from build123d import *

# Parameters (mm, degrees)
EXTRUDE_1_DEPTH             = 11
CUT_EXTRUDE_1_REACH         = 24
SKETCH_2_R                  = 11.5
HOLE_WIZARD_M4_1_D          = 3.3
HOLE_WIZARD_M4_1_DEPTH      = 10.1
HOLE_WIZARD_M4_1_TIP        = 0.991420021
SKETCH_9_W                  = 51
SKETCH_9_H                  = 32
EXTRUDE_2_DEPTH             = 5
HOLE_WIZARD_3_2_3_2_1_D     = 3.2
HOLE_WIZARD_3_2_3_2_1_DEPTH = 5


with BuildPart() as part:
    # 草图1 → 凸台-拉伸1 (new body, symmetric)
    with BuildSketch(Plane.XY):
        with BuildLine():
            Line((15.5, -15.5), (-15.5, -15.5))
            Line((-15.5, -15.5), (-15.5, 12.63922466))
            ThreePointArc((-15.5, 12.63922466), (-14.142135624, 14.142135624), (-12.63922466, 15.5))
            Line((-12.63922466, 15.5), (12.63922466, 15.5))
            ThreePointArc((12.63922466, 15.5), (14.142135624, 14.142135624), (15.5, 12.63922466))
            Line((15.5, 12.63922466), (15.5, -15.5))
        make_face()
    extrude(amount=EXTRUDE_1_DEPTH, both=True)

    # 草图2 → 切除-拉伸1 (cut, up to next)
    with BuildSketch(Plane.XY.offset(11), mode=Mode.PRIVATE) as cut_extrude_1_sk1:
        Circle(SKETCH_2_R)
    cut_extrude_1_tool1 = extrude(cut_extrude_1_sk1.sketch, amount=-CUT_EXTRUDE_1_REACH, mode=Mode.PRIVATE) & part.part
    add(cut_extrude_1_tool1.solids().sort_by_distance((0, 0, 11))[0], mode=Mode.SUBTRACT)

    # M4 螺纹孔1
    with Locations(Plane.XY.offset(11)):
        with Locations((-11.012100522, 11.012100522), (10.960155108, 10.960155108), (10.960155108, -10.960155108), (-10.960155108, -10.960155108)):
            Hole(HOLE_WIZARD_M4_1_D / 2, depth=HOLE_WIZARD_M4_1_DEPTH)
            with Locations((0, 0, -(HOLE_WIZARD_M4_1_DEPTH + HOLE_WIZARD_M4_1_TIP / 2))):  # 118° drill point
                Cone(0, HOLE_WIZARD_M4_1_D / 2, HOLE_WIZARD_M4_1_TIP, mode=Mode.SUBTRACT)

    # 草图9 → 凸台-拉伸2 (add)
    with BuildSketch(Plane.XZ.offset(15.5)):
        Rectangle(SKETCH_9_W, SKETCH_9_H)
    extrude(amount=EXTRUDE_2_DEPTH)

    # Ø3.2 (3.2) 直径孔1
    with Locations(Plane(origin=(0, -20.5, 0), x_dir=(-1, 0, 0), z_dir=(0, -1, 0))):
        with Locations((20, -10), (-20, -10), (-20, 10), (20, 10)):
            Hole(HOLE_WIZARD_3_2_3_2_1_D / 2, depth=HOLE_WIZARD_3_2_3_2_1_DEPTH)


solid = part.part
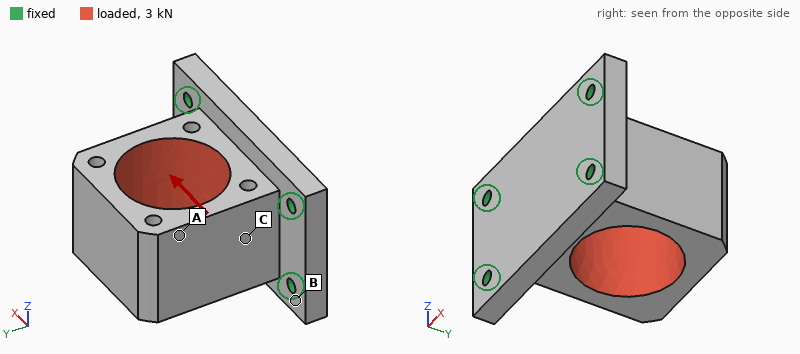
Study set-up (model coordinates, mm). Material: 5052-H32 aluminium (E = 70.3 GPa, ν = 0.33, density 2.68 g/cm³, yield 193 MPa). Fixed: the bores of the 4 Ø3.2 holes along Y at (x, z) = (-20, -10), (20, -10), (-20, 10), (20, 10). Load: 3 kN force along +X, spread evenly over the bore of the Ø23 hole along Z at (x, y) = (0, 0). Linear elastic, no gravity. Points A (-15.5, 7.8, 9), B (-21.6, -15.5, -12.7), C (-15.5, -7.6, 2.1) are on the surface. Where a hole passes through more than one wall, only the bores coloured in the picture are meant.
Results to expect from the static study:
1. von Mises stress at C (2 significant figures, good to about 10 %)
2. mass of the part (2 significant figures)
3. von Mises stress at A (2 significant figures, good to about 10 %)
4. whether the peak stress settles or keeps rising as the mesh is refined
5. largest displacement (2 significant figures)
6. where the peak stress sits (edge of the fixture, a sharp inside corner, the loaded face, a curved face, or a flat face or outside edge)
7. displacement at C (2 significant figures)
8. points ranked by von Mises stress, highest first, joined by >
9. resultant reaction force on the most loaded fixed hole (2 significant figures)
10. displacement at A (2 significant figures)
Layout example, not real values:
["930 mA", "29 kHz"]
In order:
["43 MPa", "52 g", "29 MPa", "keeps rising", "55 µm", "edge of the fixture", "14 µm", "C > A > B", "1.1 kN", "48 µm"]
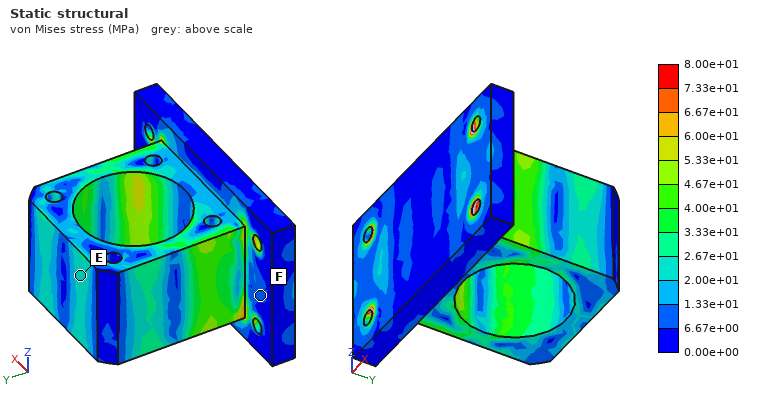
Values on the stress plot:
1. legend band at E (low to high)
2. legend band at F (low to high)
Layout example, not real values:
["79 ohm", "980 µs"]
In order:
["2.00e+01 to 2.67e+01 MPa", "6.67e+00 to 1.33e+01 MPa"]
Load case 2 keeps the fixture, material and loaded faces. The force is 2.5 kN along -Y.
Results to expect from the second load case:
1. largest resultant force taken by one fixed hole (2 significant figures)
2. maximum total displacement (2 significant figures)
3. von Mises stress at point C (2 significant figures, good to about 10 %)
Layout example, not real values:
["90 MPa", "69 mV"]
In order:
["670 N", "12 µm", "14 MPa"]
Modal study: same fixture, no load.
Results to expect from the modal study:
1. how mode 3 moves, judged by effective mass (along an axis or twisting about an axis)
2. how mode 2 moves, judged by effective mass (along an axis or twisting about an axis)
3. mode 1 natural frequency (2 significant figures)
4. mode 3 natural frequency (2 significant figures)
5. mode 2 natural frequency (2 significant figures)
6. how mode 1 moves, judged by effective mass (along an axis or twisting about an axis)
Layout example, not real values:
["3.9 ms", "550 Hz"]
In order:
["twisting about Y", "along X", "6700 Hz", "13 kHz", "7400 Hz", "along Z"]
